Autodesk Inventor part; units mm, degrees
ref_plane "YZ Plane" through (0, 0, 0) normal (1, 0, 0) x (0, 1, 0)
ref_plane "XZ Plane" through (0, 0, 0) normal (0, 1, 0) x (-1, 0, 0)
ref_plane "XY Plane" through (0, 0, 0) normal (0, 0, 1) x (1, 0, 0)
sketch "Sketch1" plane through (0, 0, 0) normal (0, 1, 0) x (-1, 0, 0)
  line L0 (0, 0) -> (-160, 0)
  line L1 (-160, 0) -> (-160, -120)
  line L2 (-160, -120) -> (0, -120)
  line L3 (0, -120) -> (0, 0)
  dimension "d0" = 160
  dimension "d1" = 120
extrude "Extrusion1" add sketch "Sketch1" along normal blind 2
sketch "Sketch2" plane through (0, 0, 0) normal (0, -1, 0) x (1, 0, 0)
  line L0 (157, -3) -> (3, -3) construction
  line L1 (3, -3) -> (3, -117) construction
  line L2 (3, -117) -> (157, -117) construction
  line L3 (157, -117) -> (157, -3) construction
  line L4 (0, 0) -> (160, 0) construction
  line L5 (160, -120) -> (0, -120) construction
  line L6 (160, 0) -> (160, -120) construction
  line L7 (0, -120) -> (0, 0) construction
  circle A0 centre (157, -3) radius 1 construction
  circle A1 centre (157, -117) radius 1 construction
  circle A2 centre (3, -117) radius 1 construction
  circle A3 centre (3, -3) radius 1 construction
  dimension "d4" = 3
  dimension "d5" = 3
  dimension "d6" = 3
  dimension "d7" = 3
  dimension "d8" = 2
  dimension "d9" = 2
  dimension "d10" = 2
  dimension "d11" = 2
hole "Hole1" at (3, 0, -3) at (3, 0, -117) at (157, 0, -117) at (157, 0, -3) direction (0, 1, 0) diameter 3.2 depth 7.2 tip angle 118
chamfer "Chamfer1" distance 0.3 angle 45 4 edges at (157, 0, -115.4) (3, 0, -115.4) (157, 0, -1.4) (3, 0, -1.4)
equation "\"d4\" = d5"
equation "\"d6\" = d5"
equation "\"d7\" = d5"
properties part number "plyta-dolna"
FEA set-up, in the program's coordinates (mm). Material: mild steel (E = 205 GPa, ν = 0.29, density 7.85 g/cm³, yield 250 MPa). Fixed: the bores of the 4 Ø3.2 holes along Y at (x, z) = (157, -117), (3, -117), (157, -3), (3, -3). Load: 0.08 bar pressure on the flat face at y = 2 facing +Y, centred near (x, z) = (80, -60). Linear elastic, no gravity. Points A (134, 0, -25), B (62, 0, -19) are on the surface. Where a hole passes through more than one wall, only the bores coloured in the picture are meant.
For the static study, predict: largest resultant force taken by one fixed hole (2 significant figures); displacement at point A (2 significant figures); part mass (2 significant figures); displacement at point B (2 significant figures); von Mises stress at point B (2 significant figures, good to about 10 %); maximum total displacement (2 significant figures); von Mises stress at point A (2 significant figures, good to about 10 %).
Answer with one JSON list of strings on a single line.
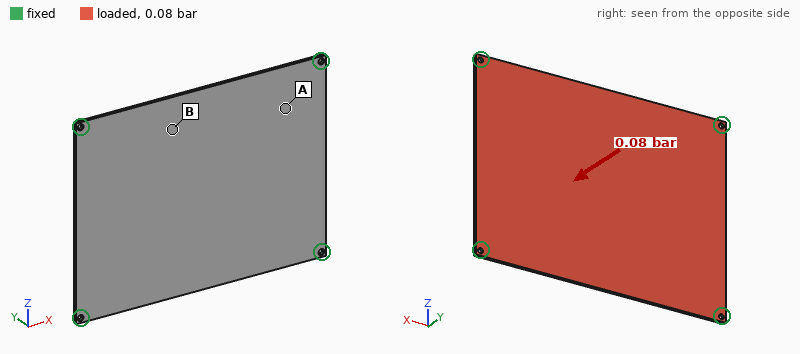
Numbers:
["39 N", "0.086 mm", "300 g", "0.17 mm", "16 MPa", "0.20 mm", "6.7 MPa"]
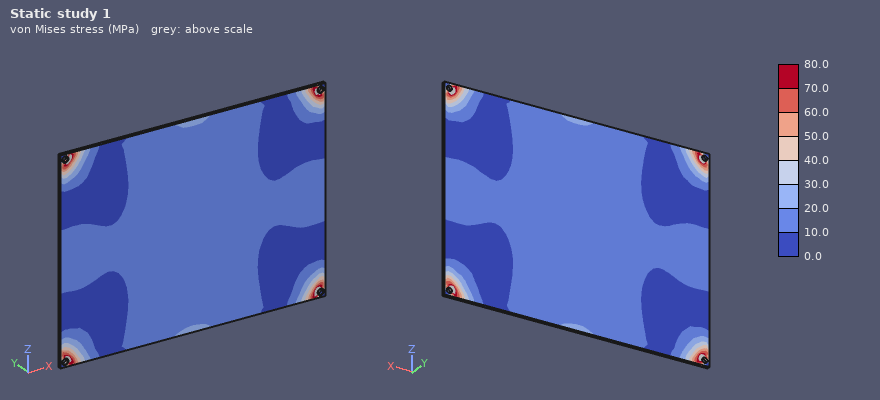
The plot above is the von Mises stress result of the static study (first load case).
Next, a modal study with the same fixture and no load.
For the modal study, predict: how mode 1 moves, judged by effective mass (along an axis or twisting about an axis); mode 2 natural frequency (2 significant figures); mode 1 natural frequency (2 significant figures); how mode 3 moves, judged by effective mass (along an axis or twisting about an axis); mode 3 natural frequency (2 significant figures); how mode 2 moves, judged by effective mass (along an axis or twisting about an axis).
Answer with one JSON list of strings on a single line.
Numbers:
["along Y", "540 Hz", "300 Hz", "twisting about Z", "690 Hz", "twisting about X"]
